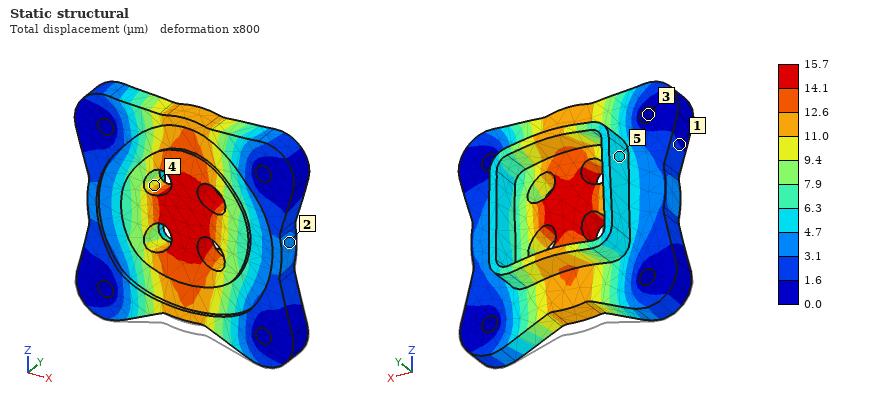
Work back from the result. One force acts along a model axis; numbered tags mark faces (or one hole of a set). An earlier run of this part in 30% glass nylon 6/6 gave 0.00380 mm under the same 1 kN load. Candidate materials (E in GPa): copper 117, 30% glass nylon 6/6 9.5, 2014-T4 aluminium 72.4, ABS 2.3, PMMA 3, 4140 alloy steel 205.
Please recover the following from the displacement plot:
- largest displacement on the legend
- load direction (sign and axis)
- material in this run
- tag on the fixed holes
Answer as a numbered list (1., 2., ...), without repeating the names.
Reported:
1. 15.7 µm
2. +Z
3. ABS
4. 3
